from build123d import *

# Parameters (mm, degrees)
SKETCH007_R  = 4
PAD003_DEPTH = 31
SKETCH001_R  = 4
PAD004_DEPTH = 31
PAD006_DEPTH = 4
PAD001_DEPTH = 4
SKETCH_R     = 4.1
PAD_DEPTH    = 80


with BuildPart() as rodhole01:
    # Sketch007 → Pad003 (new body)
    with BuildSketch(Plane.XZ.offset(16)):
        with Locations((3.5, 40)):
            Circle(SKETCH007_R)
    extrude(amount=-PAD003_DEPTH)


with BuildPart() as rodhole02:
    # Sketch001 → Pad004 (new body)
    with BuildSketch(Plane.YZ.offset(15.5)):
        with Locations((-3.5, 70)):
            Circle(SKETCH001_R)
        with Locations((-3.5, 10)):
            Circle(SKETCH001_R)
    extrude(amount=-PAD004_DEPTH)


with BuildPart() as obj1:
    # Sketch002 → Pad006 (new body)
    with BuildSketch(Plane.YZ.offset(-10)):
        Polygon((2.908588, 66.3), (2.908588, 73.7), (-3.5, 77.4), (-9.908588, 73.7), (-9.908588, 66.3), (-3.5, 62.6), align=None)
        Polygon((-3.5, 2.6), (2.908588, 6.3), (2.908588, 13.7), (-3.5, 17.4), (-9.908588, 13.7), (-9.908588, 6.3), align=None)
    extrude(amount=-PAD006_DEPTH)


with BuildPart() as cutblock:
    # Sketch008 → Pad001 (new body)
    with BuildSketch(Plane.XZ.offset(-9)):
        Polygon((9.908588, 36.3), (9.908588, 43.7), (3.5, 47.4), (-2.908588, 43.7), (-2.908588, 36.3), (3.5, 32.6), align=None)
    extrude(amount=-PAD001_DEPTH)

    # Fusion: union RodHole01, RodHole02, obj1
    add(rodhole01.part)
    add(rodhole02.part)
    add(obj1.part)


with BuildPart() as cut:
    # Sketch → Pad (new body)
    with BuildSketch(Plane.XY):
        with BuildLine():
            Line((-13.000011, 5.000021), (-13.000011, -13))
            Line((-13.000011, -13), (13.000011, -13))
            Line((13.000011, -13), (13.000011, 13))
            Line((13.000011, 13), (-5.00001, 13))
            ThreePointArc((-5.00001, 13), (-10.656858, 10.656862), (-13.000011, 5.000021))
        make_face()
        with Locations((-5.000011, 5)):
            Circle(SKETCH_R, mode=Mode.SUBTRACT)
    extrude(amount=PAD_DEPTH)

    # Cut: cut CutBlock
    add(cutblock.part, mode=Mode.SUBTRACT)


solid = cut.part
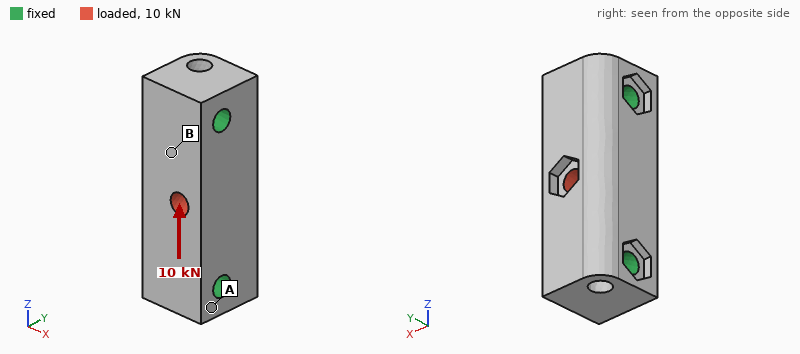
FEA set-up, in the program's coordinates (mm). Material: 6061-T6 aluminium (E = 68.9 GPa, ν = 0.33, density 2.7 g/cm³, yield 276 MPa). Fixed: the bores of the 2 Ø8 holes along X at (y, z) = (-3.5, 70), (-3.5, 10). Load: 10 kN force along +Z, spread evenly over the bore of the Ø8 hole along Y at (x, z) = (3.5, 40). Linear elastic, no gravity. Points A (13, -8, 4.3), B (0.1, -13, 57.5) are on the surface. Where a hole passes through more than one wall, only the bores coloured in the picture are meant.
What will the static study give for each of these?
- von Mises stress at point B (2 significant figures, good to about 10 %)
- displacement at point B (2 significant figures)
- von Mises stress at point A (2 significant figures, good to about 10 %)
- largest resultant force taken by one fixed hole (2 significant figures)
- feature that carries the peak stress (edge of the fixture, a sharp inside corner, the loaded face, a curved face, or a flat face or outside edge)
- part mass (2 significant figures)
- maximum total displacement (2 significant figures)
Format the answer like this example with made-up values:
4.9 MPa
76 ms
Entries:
11 MPa
1.8 µm
4.0 MPa
5.0 kN
the loaded face
120 g
6.2 µm
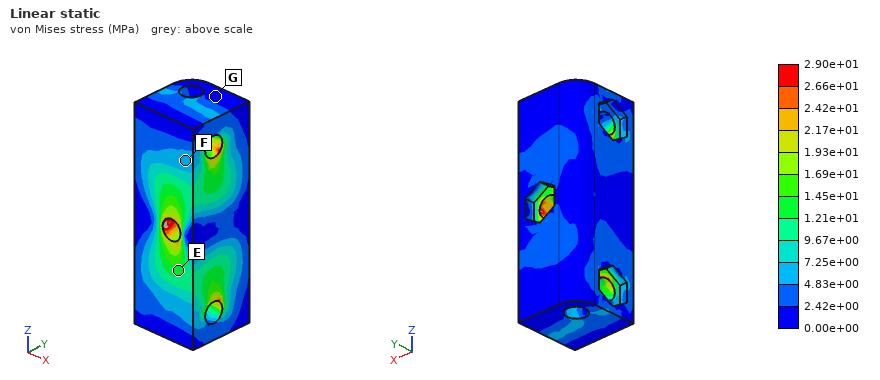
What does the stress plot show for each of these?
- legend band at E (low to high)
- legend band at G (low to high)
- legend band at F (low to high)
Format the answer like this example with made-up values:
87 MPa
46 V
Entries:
1.21e+01 to 1.45e+01 MPa
0.00e+00 to 2.42e+00 MPa
4.83e+00 to 7.25e+00 MPa
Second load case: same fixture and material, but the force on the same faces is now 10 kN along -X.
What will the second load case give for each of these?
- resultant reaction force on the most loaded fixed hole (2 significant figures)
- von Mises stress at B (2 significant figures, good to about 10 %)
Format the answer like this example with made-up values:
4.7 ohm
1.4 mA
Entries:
5.0 kN
25 MPa
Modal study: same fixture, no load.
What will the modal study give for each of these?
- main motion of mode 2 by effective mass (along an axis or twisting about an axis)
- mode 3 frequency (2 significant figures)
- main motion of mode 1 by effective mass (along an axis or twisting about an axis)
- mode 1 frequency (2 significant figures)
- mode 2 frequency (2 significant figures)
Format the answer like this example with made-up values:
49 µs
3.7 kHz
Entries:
along X
23 kHz
along Y
17 kHz
19 kHz
